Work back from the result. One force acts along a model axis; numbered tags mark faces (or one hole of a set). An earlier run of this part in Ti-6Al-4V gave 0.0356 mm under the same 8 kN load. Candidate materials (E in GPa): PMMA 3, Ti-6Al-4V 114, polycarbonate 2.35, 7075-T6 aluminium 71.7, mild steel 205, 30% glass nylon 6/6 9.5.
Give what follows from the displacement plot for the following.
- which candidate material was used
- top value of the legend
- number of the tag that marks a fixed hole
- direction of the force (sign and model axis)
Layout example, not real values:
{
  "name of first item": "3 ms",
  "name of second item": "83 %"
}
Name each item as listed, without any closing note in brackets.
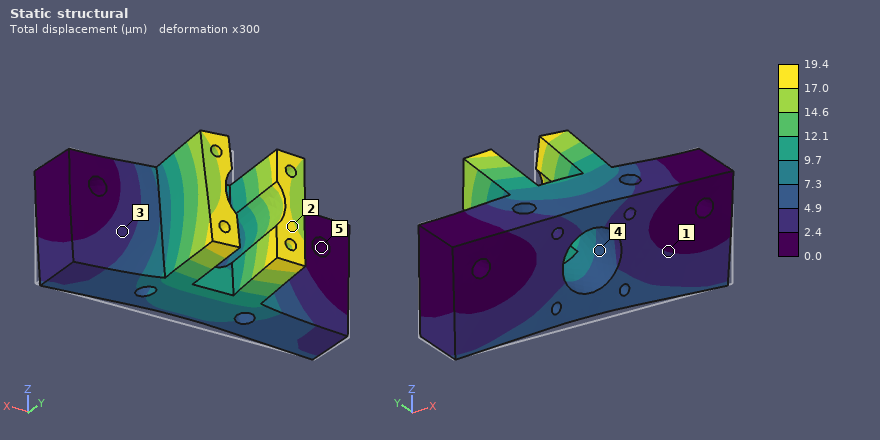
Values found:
{
  "which candidate material was used": "mild steel",
  "top value of the legend": "19.4 µm",
  "number of the tag that marks a fixed hole": "5",
  "direction of the force": "+Z"
}
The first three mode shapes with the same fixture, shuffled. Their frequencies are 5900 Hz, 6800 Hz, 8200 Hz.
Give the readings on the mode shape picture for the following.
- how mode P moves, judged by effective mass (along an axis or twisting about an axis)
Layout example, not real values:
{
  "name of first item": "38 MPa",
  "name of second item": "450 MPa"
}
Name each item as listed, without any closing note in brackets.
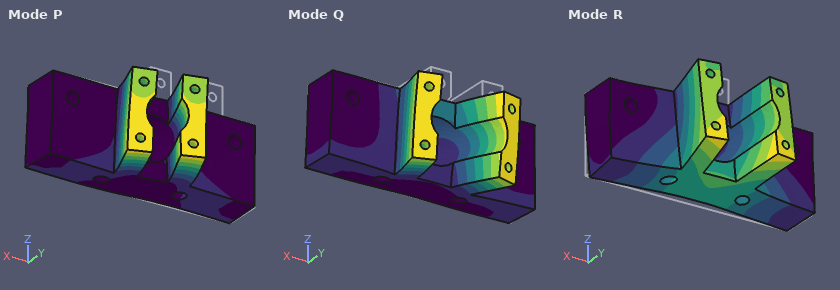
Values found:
{
  "how mode P moves, judged by effective mass": "along X"
}
